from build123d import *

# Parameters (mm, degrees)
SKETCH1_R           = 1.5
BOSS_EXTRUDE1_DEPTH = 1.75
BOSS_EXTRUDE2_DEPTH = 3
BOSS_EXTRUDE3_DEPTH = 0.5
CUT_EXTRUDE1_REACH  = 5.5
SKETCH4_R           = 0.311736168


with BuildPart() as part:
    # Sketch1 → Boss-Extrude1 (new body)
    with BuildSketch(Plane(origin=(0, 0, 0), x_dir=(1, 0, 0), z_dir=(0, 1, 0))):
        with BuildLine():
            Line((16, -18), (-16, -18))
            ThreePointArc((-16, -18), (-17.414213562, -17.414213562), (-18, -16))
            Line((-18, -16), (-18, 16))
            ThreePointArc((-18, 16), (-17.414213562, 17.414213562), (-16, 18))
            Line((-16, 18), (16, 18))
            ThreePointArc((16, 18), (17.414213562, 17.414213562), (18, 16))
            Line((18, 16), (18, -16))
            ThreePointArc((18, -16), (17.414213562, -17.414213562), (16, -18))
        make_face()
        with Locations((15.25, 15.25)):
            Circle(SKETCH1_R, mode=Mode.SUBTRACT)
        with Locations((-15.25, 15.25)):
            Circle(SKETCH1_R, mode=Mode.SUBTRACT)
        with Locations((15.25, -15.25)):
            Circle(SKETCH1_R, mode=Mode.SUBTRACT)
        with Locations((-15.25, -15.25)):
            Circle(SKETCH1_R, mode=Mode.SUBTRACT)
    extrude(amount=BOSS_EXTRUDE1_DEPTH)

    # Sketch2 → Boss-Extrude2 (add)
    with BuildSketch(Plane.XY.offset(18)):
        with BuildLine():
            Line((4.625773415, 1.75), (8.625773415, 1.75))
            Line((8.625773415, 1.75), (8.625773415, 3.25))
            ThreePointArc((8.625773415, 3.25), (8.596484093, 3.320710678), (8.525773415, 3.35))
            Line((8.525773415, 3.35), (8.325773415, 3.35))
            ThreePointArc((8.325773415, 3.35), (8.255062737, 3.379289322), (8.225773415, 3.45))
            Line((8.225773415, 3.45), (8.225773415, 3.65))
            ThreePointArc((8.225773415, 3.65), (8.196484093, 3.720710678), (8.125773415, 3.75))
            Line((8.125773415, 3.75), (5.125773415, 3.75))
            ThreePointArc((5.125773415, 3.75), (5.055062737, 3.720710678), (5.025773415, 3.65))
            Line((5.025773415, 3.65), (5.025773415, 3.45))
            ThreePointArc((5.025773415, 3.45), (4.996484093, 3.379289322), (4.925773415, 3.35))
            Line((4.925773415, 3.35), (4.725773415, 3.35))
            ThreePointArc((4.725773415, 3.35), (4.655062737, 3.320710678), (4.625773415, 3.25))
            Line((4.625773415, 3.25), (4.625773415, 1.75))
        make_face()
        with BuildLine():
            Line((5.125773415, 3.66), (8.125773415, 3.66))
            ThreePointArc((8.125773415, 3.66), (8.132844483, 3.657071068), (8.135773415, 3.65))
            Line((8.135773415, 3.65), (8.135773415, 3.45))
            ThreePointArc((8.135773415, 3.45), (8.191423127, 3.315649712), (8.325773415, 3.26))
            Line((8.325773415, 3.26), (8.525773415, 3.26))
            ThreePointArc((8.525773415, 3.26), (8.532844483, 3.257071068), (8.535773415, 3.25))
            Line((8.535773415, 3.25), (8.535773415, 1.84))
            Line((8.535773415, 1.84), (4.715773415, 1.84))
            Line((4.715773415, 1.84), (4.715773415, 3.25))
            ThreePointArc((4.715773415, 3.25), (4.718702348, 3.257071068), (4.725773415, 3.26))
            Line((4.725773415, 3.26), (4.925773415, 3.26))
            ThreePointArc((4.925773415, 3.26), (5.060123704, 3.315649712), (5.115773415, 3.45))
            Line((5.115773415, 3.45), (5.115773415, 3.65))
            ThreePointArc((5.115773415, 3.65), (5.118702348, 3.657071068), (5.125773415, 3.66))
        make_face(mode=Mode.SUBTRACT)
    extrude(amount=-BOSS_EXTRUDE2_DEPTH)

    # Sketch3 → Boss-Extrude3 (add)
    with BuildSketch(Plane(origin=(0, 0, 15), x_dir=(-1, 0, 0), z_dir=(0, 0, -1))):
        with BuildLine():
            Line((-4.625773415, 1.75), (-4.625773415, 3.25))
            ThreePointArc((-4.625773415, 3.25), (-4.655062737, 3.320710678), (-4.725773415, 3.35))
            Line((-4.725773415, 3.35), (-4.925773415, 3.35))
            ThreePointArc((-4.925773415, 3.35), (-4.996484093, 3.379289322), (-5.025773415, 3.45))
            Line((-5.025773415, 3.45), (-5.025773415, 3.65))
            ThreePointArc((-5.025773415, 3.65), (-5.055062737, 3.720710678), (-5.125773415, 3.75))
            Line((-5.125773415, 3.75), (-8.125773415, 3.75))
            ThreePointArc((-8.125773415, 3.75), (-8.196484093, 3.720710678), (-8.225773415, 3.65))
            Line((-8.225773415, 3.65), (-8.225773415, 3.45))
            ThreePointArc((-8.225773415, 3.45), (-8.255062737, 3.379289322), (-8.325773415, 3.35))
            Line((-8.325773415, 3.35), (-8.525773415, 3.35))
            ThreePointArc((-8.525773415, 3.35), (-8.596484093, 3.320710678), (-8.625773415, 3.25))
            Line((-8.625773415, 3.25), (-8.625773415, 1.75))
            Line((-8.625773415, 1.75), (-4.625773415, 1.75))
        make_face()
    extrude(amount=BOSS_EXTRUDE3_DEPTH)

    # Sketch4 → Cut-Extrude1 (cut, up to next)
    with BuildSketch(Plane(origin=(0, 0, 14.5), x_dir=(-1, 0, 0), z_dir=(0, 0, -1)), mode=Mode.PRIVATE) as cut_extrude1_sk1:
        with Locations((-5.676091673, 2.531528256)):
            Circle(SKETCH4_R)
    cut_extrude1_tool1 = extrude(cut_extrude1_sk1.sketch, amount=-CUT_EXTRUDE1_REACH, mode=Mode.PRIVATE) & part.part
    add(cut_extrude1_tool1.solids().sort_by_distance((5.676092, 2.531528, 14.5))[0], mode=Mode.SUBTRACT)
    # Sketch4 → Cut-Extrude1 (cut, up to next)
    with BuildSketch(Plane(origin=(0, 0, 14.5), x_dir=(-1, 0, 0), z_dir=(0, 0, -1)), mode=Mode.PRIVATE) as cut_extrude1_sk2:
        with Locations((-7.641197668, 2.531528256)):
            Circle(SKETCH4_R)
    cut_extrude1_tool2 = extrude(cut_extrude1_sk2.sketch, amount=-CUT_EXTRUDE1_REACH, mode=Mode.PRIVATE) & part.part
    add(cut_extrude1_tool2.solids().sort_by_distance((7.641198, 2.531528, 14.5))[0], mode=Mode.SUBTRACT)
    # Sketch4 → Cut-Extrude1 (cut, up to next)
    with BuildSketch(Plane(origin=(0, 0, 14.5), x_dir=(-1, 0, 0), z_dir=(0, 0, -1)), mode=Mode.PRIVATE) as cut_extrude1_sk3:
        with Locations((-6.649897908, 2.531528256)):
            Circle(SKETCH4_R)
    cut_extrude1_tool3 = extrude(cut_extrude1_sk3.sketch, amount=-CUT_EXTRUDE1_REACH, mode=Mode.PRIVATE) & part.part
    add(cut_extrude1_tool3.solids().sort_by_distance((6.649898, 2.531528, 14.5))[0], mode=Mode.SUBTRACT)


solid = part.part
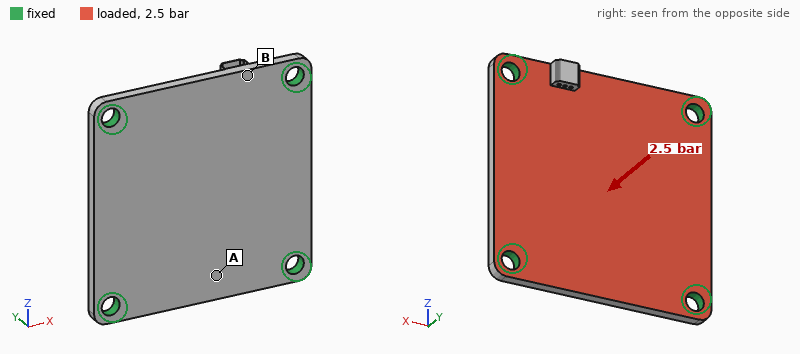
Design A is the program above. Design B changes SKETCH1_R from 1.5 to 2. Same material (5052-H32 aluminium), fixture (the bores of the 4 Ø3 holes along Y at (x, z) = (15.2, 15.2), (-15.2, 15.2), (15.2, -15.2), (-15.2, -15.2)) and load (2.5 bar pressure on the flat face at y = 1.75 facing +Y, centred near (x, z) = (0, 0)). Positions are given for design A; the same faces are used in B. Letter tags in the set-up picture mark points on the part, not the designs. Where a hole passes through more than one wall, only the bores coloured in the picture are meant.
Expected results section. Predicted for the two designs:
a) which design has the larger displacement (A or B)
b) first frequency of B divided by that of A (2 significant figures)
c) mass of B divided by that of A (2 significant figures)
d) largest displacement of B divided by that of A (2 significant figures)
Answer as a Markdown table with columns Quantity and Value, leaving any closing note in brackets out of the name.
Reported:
| Quantity | Value |
|---|---|
| which design has the larger displacement | A |
| first frequency of B divided by that of A | 1.1 |
| mass of B divided by that of A | 0.98 |
| largest displacement of B divided by that of A | 0.86 |
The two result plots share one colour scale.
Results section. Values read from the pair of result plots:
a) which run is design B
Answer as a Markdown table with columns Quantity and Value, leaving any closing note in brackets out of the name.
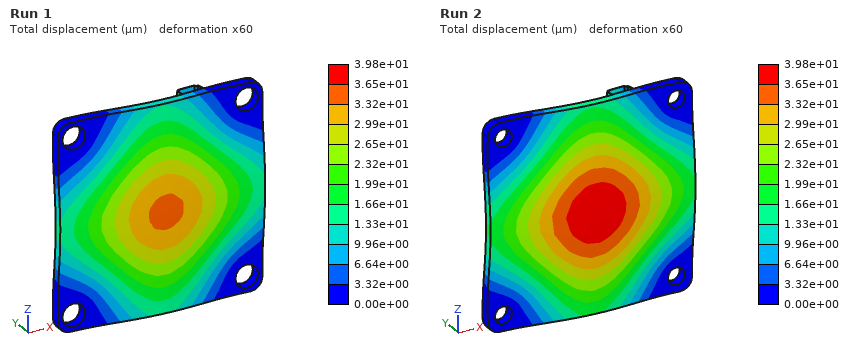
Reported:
| Quantity | Value |
|---|---|
| which run is design B | Run 1 |
